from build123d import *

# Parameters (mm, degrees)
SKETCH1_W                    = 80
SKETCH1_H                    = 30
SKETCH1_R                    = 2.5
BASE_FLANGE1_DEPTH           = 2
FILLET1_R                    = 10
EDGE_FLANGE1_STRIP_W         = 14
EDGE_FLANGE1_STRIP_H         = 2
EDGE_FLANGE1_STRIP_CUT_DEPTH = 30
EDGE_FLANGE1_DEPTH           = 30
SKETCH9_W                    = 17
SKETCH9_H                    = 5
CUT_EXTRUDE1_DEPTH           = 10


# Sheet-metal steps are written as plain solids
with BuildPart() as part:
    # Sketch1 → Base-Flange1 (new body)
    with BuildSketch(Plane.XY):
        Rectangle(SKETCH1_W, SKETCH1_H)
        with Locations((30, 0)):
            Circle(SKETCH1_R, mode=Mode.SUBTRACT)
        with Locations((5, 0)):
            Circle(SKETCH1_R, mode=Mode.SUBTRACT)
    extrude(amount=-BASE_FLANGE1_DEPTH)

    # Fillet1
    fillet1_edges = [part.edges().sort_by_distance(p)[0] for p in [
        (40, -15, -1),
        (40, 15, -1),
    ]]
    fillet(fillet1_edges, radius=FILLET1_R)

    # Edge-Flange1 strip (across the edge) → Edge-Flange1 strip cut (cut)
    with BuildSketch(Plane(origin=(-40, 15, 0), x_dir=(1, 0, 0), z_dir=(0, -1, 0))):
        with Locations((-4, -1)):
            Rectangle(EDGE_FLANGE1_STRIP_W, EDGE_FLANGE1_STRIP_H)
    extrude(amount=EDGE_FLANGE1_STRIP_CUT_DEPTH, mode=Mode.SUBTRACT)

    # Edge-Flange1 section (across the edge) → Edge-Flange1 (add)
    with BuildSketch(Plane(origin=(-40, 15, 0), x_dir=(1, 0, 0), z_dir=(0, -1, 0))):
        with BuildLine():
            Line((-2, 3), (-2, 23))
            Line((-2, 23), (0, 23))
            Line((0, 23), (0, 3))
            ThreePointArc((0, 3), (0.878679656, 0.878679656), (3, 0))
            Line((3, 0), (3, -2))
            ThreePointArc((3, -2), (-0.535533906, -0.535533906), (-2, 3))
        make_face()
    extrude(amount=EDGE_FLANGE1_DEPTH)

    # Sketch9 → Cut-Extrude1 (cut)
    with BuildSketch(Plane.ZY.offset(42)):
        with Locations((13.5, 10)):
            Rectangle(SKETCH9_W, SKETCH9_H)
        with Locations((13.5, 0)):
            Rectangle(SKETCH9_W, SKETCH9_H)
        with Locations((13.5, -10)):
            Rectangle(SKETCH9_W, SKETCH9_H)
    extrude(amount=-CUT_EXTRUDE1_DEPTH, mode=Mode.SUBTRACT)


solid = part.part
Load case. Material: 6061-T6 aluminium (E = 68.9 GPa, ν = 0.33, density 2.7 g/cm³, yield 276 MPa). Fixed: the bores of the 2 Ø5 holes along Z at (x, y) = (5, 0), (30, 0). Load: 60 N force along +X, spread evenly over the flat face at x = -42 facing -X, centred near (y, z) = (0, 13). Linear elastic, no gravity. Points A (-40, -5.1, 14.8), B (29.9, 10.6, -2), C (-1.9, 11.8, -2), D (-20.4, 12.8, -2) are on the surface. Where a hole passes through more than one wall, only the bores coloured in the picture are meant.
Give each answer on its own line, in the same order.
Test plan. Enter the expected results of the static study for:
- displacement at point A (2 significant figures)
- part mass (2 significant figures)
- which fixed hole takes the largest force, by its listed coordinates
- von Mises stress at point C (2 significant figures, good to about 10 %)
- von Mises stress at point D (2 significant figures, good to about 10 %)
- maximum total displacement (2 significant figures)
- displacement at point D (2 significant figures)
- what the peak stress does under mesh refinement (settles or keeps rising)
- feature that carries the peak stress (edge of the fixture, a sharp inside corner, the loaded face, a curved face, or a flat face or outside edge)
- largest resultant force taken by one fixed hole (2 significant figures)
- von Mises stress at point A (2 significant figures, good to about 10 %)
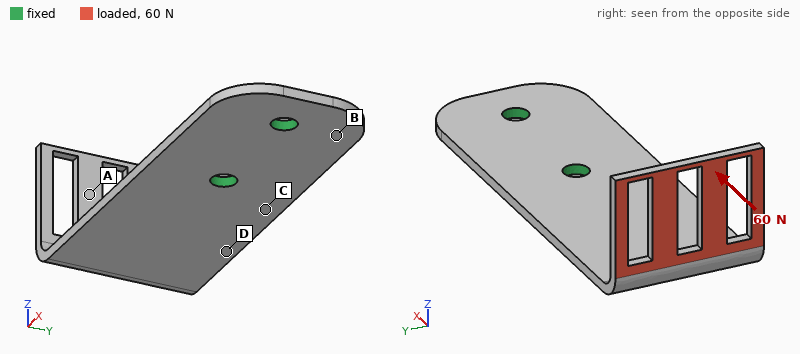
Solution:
0.73 mm
15 g
(5, 0)
35 MPa
41 MPa
0.96 mm
0.17 mm
keeps rising
edge of the fixture
48 N
11 MPa
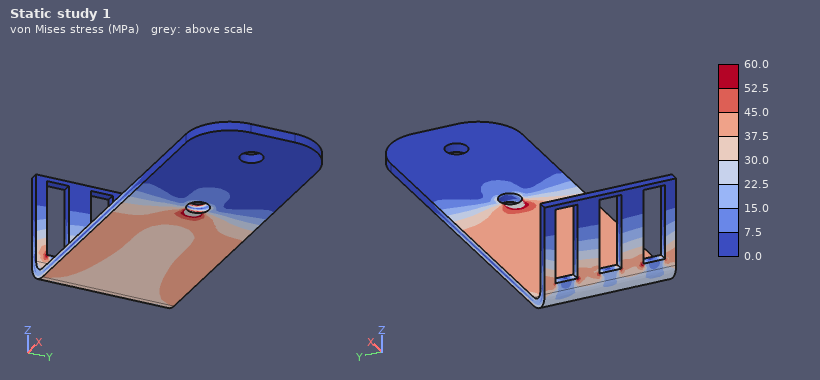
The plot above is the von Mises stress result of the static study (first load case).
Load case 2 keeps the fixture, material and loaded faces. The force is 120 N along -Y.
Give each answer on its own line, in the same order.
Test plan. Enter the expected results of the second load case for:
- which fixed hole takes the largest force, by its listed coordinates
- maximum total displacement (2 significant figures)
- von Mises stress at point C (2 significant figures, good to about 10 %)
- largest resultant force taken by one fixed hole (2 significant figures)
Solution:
(5, 0)
0.99 mm
56 MPa
290 N
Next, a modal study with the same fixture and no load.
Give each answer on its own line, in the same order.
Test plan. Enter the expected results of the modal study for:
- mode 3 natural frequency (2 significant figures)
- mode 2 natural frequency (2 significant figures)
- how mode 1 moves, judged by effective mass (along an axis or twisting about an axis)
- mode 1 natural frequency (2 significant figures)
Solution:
2000 Hz
1200 Hz
along Z
510 Hz
